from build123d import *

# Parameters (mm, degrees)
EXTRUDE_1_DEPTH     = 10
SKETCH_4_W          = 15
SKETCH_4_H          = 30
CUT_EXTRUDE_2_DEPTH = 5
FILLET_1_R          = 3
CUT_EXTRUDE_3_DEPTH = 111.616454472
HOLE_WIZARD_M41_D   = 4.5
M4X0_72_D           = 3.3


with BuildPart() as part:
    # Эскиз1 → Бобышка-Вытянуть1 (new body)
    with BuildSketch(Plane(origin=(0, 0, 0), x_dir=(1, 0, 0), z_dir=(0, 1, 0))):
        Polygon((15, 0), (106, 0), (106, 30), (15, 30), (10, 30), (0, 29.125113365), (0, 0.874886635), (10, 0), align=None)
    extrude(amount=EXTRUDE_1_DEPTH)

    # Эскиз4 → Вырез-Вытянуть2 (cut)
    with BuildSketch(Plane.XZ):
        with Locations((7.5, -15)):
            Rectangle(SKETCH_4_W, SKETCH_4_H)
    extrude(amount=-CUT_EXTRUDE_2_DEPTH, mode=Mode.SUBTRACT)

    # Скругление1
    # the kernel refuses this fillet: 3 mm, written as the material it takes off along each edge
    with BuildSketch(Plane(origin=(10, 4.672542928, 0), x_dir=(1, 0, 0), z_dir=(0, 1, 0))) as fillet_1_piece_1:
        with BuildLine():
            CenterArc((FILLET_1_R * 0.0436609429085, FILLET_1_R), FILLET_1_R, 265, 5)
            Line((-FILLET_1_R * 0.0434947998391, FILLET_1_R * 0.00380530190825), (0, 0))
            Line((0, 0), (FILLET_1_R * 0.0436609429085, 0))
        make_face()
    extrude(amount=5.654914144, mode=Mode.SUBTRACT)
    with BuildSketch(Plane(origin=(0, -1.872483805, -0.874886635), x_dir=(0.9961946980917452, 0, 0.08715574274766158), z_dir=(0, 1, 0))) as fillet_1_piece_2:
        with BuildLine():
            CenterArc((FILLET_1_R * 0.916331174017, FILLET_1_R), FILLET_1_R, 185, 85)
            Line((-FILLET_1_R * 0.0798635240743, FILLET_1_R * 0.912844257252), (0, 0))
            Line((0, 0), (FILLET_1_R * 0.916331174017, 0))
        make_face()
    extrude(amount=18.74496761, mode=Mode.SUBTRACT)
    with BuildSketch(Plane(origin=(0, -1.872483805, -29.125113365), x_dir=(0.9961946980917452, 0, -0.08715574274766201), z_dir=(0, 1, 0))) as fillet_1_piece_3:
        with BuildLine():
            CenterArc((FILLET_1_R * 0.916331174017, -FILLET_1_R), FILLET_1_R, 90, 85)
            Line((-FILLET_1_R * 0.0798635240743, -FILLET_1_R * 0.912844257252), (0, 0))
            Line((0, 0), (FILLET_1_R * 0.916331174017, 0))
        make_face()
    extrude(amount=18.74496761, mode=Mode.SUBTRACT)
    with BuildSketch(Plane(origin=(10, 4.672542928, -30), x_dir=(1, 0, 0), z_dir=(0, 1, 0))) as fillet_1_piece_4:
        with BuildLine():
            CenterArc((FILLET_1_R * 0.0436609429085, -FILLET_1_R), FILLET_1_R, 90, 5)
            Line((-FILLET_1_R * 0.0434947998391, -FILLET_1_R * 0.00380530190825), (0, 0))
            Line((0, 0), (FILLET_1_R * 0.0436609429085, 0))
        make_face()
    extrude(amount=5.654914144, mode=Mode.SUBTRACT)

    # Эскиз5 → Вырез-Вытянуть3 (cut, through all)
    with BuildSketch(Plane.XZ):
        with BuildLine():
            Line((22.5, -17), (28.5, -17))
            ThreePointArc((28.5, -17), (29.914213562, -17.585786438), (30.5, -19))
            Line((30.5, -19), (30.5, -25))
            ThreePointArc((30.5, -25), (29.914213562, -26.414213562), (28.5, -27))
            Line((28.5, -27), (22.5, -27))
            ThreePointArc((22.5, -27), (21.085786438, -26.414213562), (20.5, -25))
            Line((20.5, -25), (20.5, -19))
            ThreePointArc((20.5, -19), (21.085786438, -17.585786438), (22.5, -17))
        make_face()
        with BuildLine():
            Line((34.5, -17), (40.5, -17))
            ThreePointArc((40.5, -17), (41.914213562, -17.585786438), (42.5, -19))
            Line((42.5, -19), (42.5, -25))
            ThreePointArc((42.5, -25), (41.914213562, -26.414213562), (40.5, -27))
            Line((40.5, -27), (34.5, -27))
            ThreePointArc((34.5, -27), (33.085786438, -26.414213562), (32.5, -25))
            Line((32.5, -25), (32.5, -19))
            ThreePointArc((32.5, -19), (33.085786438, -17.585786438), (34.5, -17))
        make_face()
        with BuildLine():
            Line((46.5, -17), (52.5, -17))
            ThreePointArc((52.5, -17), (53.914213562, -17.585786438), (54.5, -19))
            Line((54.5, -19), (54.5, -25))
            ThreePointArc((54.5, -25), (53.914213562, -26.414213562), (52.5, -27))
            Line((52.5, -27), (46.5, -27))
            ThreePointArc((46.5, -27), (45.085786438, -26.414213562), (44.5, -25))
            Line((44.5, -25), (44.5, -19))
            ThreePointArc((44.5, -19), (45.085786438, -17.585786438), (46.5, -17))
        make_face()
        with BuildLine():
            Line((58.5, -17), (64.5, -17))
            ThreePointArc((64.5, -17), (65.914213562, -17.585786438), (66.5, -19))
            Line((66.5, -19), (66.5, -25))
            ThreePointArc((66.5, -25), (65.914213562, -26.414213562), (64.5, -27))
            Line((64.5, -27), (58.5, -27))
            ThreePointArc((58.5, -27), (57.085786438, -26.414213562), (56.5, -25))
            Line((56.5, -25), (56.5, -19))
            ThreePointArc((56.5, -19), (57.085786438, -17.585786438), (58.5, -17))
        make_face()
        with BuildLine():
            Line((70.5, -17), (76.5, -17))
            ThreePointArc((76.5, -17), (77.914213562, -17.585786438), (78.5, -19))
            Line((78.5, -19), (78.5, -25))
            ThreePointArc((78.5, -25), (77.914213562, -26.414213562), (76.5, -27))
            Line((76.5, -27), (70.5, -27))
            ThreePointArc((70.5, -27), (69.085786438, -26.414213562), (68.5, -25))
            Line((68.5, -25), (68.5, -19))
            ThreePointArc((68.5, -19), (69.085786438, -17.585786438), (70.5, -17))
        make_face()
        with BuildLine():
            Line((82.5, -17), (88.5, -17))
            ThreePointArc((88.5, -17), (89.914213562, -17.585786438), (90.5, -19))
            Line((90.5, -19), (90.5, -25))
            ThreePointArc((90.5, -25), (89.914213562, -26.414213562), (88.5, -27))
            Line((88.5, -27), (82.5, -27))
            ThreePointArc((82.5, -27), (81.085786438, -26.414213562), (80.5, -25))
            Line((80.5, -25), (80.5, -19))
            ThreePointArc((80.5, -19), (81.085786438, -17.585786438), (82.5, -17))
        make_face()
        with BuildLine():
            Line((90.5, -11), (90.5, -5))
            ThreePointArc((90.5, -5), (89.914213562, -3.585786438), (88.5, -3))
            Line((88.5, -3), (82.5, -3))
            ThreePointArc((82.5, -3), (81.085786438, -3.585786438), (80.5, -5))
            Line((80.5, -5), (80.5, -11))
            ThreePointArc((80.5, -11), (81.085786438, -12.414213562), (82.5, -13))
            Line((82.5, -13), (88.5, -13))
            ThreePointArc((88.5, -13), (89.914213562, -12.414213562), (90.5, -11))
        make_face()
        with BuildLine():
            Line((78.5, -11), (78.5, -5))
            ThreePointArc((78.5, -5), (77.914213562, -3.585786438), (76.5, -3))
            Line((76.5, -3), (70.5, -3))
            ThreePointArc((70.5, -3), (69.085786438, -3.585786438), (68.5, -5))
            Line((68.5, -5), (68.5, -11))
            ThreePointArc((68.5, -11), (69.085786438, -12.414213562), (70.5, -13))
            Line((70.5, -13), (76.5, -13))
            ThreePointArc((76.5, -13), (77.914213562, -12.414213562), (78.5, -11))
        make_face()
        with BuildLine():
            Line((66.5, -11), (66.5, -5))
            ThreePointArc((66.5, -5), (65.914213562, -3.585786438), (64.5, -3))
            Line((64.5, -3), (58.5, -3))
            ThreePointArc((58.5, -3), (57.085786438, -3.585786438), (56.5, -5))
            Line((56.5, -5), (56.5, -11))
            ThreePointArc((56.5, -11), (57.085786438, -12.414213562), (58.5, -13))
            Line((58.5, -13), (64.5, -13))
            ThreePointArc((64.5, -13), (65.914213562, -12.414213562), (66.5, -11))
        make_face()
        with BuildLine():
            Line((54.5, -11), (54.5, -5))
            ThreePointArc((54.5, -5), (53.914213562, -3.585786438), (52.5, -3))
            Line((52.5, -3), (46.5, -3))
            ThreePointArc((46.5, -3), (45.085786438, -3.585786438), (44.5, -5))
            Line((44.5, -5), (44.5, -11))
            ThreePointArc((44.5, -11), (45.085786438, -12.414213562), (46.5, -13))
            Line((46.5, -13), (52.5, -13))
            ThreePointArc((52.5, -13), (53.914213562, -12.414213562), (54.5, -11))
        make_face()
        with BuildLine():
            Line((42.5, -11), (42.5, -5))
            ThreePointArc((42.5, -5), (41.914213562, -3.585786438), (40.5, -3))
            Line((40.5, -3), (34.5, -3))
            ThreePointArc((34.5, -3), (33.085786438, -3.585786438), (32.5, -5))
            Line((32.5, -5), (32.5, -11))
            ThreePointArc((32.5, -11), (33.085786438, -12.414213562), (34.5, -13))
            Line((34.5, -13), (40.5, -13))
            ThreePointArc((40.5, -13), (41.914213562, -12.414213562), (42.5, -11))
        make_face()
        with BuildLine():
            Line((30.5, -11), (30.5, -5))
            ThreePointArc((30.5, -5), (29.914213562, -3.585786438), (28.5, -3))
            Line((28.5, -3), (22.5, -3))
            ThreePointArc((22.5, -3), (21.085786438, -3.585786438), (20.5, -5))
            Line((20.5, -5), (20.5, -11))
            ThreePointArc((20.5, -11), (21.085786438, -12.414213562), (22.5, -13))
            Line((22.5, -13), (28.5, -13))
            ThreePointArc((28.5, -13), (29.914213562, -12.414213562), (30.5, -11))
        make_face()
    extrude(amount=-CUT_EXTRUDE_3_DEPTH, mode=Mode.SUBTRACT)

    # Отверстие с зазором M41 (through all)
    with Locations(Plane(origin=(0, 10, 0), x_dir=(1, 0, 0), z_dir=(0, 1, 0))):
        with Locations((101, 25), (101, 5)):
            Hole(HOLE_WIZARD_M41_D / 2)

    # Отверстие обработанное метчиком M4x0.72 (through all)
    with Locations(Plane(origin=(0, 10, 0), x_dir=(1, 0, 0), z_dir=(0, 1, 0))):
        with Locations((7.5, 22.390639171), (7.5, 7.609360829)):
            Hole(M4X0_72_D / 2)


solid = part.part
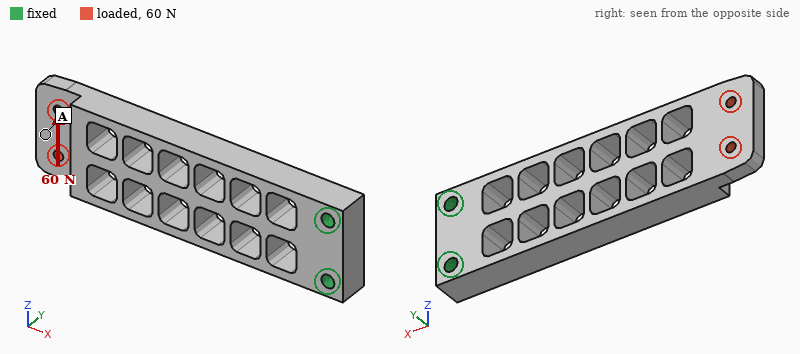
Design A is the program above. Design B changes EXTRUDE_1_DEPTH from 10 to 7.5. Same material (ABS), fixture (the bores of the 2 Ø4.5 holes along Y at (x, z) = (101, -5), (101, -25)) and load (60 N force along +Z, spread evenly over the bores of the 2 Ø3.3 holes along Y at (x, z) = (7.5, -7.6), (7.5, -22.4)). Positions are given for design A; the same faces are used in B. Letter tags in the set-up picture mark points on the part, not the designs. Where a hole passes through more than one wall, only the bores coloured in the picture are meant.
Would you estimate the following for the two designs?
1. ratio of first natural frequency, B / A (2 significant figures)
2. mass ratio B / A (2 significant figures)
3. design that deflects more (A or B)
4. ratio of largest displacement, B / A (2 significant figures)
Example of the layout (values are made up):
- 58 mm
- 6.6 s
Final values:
- 0.82
- 0.72
- B
- 1.4
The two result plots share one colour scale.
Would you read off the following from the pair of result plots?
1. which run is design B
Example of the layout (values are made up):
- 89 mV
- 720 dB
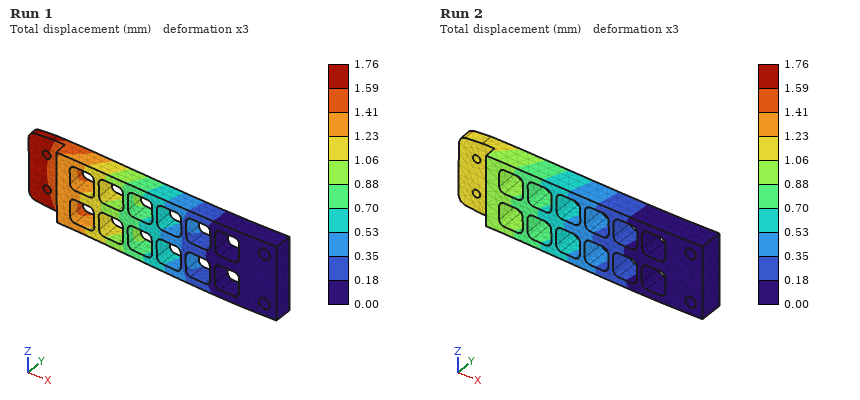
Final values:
- Run 1
